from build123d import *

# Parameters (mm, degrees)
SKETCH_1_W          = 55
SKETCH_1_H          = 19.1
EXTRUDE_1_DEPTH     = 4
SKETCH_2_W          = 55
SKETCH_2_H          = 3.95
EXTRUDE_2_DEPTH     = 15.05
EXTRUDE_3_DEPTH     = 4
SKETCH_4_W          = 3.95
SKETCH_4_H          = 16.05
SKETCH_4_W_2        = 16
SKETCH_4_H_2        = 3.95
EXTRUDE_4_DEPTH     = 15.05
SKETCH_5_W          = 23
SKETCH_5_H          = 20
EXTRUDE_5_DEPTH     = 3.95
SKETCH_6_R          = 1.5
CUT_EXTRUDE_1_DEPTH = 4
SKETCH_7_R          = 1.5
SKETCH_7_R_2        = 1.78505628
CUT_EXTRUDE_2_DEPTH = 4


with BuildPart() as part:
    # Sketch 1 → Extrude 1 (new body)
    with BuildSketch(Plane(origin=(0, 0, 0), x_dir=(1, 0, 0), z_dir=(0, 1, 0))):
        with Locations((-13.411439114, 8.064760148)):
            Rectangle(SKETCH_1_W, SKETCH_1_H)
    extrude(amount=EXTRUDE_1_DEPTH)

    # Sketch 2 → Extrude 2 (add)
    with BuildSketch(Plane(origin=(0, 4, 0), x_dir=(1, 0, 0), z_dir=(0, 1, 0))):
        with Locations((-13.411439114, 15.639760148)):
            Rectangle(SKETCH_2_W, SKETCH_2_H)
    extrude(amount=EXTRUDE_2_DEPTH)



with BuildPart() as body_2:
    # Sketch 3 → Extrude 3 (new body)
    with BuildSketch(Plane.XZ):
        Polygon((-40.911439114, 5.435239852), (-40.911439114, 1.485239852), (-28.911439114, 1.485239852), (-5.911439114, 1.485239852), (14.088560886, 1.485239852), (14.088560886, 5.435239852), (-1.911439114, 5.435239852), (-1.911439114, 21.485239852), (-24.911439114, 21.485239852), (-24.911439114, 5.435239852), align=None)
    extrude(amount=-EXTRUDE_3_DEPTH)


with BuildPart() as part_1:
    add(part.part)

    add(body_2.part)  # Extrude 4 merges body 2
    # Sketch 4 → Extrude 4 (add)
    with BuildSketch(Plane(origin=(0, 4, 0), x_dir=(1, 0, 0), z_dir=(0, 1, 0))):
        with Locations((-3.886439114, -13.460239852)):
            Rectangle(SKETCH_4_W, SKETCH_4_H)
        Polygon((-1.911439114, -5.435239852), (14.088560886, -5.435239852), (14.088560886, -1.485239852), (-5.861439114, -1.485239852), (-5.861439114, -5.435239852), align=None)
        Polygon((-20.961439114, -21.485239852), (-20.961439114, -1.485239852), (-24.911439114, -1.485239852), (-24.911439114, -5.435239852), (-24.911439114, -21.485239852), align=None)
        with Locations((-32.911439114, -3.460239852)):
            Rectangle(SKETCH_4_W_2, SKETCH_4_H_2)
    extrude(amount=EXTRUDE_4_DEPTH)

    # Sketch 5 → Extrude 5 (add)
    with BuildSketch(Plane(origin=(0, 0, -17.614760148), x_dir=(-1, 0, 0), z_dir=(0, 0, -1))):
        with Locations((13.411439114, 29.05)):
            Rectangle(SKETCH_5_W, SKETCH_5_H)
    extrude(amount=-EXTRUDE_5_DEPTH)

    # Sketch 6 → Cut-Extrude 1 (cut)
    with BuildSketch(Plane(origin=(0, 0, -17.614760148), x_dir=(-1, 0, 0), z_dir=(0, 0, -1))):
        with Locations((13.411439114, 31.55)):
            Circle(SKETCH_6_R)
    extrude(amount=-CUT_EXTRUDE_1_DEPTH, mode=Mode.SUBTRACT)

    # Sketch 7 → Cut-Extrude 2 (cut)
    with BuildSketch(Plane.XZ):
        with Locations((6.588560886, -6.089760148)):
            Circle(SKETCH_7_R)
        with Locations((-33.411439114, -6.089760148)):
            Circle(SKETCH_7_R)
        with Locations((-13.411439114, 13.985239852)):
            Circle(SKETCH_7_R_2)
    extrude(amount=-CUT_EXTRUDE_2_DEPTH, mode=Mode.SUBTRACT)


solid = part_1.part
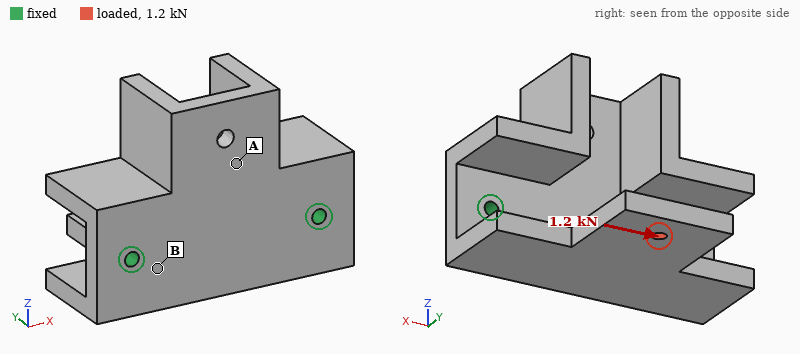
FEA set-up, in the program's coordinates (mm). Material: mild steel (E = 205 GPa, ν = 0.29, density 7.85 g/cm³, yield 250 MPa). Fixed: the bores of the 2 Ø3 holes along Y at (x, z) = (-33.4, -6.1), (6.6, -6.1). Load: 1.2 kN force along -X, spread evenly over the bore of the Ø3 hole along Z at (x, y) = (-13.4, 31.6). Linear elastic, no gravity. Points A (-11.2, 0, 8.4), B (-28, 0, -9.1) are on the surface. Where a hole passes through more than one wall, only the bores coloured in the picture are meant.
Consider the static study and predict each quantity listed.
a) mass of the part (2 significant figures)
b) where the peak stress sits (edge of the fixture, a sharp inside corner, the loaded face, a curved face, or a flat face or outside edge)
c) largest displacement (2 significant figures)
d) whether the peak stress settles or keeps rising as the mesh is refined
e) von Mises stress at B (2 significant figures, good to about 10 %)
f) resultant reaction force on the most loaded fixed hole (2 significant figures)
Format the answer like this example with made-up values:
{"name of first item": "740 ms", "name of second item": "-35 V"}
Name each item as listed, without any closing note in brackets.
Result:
{"mass of the part": "120 g", "where the peak stress sits": "edge of the fixture", "largest displacement": "35 µm", "whether the peak stress settles or keeps rising as the mesh is refined": "keeps rising", "von Mises stress at B": "37 MPa", "resultant reaction force on the most loaded fixed hole": "1.1 kN"}
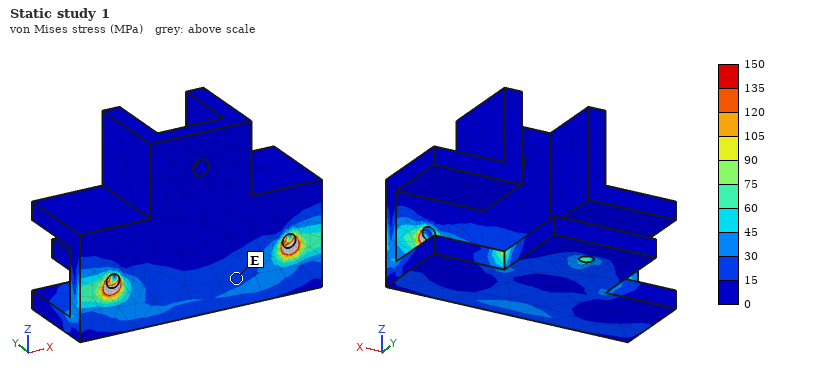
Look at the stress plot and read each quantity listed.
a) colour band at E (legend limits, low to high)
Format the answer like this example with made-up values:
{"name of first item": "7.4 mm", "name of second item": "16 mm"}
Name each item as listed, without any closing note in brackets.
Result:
{"colour band at E": "15 to 30 MPa"}
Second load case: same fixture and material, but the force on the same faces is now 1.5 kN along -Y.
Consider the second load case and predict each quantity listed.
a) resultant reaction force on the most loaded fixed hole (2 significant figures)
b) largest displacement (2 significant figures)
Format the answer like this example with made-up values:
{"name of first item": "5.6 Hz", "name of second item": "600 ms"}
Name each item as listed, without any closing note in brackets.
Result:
{"resultant reaction force on the most loaded fixed hole": "790 N", "largest displacement": "68 µm"}
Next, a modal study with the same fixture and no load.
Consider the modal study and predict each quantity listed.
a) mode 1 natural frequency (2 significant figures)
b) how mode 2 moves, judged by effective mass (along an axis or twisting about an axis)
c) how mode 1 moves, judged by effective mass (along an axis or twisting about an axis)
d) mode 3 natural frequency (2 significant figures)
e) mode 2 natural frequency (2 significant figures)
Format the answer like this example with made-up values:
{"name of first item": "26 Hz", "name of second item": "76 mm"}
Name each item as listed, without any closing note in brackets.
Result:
{"mode 1 natural frequency": "2100 Hz", "how mode 2 moves, judged by effective mass": "along Y", "how mode 1 moves, judged by effective mass": "along Z", "mode 3 natural frequency": "6400 Hz", "mode 2 natural frequency": "3000 Hz"}
